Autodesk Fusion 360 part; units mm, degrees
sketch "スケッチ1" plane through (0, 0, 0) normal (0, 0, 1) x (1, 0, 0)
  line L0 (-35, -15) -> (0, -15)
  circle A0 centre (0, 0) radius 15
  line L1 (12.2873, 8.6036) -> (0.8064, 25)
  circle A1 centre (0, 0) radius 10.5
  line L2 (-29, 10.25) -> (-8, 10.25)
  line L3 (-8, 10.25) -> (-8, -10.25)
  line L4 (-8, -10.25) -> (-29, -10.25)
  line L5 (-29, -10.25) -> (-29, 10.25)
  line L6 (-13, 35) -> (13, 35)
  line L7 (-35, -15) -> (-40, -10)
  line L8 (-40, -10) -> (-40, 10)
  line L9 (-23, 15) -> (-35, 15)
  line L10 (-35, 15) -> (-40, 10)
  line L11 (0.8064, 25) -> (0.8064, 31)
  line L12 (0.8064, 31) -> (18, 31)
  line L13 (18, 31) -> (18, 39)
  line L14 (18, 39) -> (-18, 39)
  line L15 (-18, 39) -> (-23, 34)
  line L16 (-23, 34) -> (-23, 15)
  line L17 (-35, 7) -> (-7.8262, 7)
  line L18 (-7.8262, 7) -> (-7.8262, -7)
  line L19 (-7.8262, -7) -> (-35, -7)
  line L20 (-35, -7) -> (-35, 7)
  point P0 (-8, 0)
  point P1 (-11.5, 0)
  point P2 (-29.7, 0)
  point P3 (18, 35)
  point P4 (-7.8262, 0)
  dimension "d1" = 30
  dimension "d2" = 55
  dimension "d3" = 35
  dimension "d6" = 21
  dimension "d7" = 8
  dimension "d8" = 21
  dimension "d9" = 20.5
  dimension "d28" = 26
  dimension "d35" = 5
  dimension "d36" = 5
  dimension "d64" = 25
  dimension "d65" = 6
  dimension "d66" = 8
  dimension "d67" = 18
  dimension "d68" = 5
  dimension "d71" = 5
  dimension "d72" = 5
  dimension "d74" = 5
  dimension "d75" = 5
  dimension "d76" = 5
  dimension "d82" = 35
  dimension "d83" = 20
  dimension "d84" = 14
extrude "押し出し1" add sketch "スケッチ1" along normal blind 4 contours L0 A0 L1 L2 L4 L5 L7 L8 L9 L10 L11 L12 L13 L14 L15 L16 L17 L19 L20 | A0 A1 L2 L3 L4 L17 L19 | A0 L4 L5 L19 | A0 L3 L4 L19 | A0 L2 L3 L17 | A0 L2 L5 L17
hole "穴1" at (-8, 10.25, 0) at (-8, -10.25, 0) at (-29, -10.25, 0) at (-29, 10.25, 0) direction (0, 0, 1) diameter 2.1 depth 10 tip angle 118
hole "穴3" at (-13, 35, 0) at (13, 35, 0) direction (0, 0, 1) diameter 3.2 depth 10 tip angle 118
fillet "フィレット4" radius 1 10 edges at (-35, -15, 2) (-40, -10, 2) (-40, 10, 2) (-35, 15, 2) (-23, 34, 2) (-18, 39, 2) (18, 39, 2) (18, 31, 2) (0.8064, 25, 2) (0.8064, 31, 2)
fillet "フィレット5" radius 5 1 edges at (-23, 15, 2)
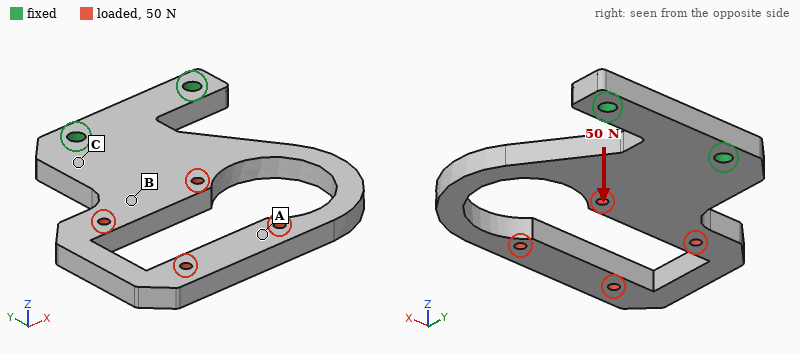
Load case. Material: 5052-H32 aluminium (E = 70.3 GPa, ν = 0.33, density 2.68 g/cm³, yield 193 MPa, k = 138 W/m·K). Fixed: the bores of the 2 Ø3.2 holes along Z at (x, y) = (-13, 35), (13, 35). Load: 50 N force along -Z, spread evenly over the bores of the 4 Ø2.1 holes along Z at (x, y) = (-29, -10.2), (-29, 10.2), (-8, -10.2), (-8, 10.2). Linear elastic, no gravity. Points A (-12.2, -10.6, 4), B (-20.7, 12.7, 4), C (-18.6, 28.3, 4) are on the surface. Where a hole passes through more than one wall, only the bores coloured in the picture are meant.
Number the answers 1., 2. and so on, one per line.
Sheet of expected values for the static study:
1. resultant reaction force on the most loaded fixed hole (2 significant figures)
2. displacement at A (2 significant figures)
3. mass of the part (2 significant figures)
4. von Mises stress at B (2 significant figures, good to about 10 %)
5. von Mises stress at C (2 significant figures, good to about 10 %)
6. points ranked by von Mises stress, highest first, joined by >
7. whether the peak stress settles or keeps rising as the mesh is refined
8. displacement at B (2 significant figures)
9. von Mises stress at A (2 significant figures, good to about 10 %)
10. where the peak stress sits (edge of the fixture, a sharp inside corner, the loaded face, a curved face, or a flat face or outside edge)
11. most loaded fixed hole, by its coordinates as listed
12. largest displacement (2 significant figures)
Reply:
1. 64 N
2. 0.18 mm
3. 17 g
4. 14 MPa
5. 21 MPa
6. C > B > A
7. keeps rising
8. 0.048 mm
9. 5.5 MPa
10. edge of the fixture
11. (-13, 35)
12. 0.22 mm
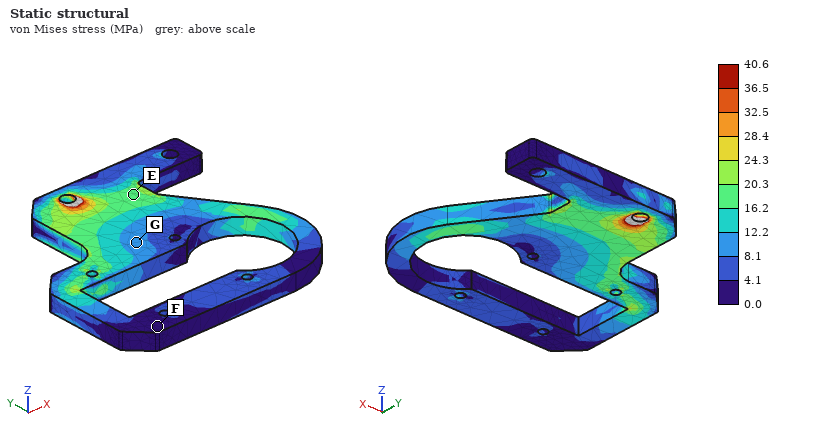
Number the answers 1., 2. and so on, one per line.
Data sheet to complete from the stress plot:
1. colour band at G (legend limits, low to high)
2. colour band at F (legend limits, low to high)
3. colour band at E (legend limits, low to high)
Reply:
1. 8.1 to 12.2 MPa
2. 0.0 to 4.1 MPa
3. 16.2 to 20.3 MPa
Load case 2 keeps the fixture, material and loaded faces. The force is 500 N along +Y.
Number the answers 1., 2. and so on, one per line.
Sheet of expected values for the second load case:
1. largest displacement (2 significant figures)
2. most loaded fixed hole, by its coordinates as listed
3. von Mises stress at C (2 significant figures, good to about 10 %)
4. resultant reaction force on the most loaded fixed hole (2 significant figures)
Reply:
1. 67 µm
2. (-13, 35)
3. 13 MPa
4. 580 N
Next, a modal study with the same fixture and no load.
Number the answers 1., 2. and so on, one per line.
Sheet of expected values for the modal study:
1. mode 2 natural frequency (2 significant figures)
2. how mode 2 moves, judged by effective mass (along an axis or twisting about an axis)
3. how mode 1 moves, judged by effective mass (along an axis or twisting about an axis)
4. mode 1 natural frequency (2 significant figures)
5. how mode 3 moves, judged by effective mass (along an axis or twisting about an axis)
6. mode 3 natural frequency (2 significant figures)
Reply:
1. 2000 Hz
2. twisting about Y
3. along Z
4. 980 Hz
5. along X
6. 2800 Hz
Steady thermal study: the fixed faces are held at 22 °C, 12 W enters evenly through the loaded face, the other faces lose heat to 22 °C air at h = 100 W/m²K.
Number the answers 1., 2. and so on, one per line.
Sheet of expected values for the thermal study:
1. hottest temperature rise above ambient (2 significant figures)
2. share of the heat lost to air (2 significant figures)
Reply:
1. 32 K
2. 52 %
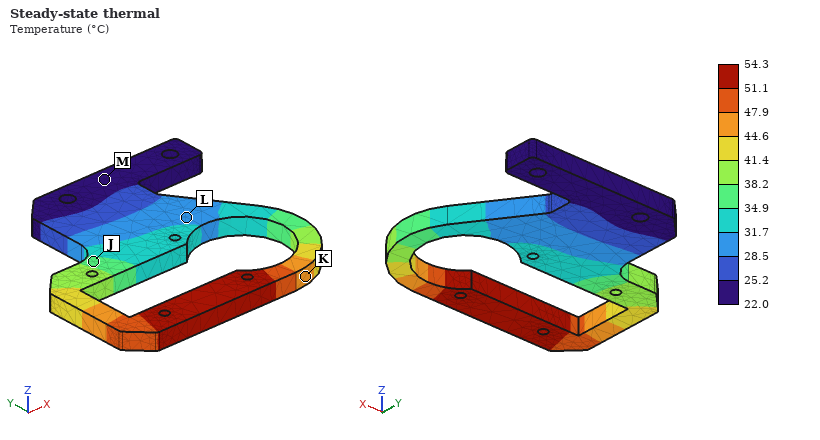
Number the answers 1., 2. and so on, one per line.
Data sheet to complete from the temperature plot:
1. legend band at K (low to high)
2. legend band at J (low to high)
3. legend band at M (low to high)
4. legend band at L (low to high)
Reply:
1. 44.6 to 47.9 °C
2. 34.9 to 38.2 °C
3. 22.0 to 25.2 °C
4. 28.5 to 31.7 °C
